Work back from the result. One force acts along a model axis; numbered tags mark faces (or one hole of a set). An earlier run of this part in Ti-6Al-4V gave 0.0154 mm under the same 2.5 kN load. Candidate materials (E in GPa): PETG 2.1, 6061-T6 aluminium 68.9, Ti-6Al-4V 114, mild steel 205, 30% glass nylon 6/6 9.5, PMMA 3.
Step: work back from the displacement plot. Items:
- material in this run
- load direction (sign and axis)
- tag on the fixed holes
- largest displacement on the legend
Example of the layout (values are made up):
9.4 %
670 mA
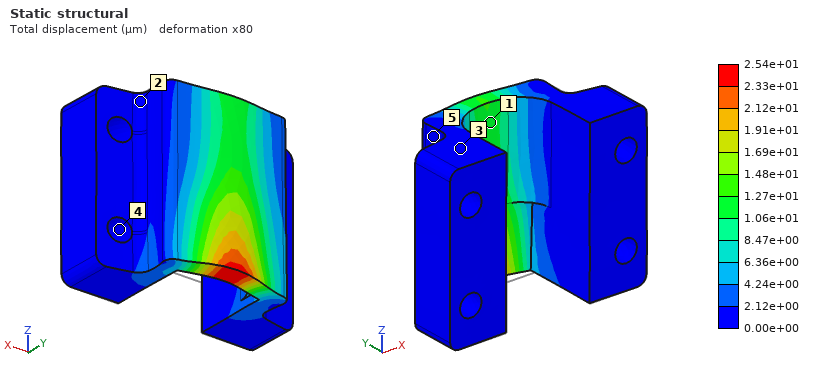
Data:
6061-T6 aluminium
+Y
4
2.54e+01 µm
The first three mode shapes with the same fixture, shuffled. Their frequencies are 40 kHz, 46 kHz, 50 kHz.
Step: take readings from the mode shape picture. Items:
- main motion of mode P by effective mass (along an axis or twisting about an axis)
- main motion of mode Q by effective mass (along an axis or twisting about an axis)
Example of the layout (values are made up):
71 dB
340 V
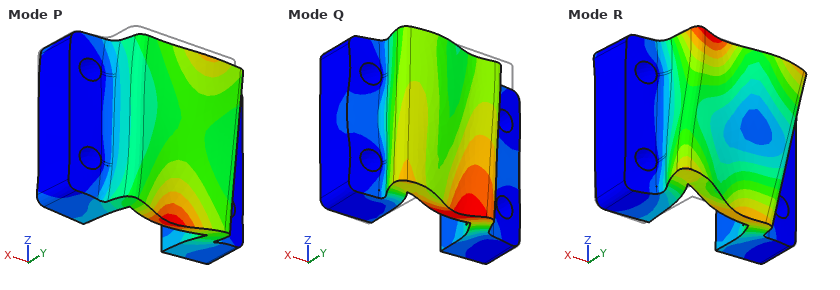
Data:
along Z
along X
